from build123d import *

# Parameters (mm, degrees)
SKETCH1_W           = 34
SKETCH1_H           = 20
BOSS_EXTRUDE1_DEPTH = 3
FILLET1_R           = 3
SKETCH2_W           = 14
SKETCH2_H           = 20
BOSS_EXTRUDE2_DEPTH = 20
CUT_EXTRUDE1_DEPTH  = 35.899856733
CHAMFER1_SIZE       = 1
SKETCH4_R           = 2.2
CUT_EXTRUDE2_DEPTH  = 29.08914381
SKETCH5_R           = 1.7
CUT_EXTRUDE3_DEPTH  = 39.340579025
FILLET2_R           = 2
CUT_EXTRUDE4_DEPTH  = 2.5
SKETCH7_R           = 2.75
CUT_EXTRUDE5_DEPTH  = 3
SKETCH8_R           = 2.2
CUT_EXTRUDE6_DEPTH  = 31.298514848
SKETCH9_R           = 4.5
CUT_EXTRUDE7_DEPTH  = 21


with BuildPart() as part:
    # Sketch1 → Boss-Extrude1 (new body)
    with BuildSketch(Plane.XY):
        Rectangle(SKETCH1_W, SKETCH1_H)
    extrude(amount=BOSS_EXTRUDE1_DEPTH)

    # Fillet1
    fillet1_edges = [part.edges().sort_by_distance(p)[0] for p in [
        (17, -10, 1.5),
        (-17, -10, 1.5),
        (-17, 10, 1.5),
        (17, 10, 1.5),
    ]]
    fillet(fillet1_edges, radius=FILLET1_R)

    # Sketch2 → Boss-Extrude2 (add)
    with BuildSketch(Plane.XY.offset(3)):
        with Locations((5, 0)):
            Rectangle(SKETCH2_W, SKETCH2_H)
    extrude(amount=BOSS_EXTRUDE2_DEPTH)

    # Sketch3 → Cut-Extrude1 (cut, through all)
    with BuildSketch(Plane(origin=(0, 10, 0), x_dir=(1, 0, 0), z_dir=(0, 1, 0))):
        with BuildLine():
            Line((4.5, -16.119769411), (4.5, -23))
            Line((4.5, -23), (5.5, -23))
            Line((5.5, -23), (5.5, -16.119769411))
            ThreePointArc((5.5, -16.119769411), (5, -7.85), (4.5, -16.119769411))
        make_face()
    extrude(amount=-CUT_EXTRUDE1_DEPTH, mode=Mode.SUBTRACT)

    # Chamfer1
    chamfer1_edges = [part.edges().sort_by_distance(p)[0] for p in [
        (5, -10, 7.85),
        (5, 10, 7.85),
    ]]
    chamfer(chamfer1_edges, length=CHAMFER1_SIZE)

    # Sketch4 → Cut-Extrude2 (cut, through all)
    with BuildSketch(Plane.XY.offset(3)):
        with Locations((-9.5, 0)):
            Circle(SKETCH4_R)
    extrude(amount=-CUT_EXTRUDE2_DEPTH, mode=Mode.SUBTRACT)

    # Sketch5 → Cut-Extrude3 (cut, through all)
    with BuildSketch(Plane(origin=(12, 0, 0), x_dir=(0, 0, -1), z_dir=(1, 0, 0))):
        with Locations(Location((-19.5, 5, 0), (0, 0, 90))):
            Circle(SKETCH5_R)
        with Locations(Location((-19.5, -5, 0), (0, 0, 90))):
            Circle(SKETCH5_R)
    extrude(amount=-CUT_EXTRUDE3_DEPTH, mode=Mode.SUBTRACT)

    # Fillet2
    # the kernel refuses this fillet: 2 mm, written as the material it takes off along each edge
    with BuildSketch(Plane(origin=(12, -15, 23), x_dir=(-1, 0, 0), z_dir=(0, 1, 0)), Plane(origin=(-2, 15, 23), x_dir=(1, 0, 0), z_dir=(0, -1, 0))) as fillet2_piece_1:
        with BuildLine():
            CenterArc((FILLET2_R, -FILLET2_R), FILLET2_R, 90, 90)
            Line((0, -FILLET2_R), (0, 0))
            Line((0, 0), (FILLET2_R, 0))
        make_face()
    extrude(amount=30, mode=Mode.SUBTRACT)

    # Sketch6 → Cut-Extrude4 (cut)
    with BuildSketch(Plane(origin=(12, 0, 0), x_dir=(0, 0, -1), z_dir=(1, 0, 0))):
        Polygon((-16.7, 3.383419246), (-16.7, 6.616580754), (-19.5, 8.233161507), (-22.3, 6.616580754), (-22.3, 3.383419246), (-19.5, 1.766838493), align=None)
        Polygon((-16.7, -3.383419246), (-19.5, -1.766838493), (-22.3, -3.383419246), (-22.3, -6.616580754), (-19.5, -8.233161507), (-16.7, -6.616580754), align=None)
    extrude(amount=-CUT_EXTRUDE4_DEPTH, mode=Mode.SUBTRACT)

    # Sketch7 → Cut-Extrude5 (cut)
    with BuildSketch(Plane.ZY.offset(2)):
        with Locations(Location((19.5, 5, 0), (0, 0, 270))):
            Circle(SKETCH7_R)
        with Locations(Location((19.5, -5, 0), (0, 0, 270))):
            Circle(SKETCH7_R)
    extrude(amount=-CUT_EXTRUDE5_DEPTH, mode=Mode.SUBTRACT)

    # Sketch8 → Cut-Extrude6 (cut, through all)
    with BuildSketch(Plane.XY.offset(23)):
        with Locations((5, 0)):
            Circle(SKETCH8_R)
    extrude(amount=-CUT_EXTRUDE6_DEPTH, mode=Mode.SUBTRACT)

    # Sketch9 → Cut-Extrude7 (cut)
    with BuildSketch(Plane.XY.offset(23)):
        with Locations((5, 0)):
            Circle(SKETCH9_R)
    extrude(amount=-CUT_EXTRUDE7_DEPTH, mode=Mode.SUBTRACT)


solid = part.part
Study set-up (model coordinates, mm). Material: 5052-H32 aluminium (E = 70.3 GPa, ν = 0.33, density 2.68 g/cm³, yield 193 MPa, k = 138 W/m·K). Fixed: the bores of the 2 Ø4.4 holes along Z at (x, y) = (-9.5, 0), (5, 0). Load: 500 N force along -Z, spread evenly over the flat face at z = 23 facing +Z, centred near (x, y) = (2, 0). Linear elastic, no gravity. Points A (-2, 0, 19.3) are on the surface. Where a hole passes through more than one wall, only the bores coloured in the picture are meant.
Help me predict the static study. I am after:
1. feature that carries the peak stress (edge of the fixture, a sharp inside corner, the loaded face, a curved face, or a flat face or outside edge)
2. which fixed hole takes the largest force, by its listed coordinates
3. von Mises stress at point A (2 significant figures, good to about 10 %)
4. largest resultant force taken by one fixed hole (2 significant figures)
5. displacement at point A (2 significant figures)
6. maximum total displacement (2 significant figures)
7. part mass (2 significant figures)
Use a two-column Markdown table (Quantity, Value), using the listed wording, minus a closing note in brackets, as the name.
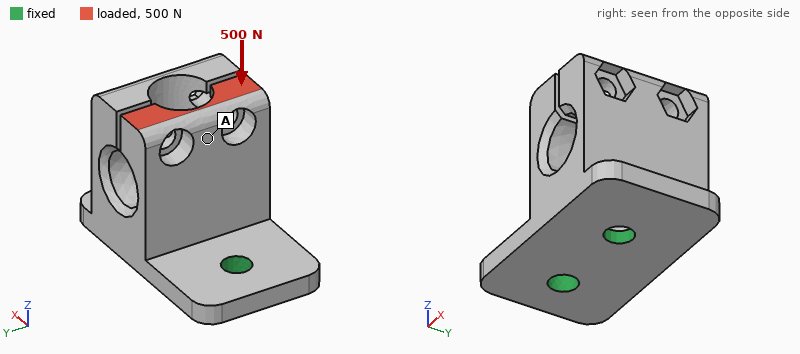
| Quantity | Value |
|---|---|
| feature that carries the peak stress | a curved face |
| which fixed hole takes the largest force, by its listed coordinates | (5, 0) |
| von Mises stress at point A | 11 MPa |
| largest resultant force taken by one fixed hole | 380 N |
| displacement at point A | 22 µm |
| maximum total displacement | 42 µm |
| part mass | 13 g |
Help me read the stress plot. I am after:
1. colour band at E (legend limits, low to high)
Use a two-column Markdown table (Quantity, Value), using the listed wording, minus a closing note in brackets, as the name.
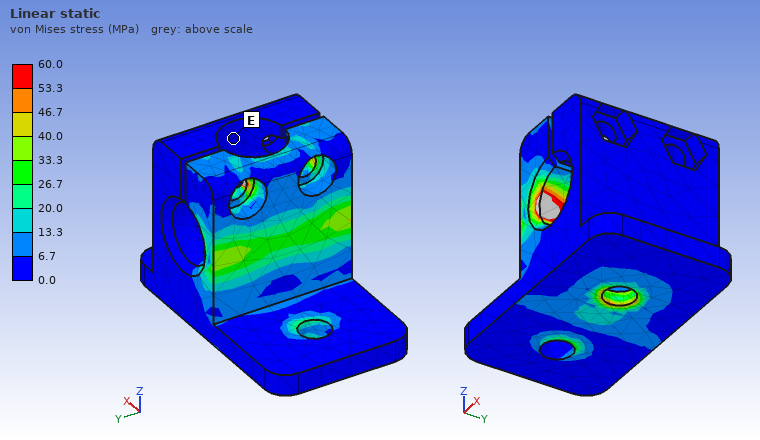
| Quantity | Value |
|---|---|
| colour band at E | 0.0 to 6.7 MPa |
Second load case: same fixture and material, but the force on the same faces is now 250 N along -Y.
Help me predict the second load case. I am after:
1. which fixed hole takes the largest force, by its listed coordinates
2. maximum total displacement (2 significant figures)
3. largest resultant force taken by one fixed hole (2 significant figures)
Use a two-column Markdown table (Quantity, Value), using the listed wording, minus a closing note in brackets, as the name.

| Quantity | Value |
|---|---|
| which fixed hole takes the largest force, by its listed coordinates | (5, 0) |
| maximum total displacement | 73 µm |
| largest resultant force taken by one fixed hole | 140 N |
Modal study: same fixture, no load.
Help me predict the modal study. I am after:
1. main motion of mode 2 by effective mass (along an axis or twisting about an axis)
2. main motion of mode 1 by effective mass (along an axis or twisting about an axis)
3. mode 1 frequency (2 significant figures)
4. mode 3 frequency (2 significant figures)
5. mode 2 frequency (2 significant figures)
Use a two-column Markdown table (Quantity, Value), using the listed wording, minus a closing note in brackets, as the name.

| Quantity | Value |
|---|---|
| main motion of mode 2 by effective mass | along X |
| main motion of mode 1 by effective mass | along Y |
| mode 1 frequency | 5400 Hz |
| mode 3 frequency | 8800 Hz |
| mode 2 frequency | 6500 Hz |
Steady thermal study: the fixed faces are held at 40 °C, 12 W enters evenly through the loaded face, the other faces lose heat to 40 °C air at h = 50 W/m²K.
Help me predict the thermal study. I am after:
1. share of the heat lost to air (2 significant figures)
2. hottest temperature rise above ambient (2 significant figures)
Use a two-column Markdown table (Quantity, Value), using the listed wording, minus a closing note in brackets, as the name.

| Quantity | Value |
|---|---|
| share of the heat lost to air | 12 % |
| hottest temperature rise above ambient | 33 K |
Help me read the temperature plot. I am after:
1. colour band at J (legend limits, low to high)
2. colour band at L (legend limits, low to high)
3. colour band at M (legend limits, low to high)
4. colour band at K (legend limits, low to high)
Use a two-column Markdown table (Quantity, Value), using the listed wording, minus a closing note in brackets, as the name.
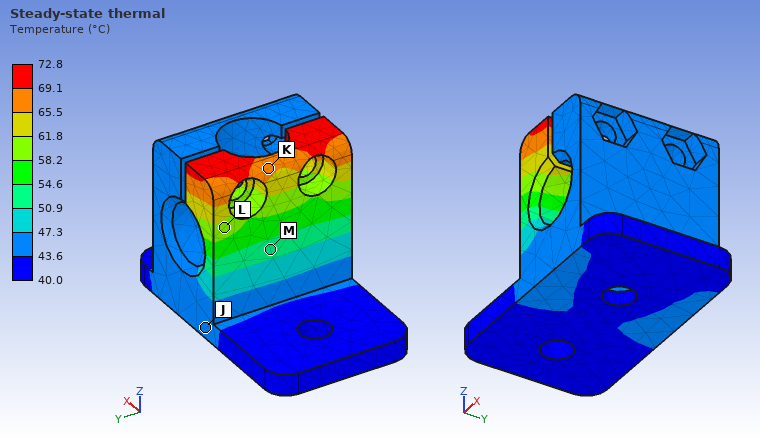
| Quantity | Value |
|---|---|
| colour band at J | 43.6 to 47.3 °C |
| colour band at L | 58.2 to 61.8 °C |
| colour band at M | 50.9 to 54.6 °C |
| colour band at K | 65.5 to 69.1 °C |
